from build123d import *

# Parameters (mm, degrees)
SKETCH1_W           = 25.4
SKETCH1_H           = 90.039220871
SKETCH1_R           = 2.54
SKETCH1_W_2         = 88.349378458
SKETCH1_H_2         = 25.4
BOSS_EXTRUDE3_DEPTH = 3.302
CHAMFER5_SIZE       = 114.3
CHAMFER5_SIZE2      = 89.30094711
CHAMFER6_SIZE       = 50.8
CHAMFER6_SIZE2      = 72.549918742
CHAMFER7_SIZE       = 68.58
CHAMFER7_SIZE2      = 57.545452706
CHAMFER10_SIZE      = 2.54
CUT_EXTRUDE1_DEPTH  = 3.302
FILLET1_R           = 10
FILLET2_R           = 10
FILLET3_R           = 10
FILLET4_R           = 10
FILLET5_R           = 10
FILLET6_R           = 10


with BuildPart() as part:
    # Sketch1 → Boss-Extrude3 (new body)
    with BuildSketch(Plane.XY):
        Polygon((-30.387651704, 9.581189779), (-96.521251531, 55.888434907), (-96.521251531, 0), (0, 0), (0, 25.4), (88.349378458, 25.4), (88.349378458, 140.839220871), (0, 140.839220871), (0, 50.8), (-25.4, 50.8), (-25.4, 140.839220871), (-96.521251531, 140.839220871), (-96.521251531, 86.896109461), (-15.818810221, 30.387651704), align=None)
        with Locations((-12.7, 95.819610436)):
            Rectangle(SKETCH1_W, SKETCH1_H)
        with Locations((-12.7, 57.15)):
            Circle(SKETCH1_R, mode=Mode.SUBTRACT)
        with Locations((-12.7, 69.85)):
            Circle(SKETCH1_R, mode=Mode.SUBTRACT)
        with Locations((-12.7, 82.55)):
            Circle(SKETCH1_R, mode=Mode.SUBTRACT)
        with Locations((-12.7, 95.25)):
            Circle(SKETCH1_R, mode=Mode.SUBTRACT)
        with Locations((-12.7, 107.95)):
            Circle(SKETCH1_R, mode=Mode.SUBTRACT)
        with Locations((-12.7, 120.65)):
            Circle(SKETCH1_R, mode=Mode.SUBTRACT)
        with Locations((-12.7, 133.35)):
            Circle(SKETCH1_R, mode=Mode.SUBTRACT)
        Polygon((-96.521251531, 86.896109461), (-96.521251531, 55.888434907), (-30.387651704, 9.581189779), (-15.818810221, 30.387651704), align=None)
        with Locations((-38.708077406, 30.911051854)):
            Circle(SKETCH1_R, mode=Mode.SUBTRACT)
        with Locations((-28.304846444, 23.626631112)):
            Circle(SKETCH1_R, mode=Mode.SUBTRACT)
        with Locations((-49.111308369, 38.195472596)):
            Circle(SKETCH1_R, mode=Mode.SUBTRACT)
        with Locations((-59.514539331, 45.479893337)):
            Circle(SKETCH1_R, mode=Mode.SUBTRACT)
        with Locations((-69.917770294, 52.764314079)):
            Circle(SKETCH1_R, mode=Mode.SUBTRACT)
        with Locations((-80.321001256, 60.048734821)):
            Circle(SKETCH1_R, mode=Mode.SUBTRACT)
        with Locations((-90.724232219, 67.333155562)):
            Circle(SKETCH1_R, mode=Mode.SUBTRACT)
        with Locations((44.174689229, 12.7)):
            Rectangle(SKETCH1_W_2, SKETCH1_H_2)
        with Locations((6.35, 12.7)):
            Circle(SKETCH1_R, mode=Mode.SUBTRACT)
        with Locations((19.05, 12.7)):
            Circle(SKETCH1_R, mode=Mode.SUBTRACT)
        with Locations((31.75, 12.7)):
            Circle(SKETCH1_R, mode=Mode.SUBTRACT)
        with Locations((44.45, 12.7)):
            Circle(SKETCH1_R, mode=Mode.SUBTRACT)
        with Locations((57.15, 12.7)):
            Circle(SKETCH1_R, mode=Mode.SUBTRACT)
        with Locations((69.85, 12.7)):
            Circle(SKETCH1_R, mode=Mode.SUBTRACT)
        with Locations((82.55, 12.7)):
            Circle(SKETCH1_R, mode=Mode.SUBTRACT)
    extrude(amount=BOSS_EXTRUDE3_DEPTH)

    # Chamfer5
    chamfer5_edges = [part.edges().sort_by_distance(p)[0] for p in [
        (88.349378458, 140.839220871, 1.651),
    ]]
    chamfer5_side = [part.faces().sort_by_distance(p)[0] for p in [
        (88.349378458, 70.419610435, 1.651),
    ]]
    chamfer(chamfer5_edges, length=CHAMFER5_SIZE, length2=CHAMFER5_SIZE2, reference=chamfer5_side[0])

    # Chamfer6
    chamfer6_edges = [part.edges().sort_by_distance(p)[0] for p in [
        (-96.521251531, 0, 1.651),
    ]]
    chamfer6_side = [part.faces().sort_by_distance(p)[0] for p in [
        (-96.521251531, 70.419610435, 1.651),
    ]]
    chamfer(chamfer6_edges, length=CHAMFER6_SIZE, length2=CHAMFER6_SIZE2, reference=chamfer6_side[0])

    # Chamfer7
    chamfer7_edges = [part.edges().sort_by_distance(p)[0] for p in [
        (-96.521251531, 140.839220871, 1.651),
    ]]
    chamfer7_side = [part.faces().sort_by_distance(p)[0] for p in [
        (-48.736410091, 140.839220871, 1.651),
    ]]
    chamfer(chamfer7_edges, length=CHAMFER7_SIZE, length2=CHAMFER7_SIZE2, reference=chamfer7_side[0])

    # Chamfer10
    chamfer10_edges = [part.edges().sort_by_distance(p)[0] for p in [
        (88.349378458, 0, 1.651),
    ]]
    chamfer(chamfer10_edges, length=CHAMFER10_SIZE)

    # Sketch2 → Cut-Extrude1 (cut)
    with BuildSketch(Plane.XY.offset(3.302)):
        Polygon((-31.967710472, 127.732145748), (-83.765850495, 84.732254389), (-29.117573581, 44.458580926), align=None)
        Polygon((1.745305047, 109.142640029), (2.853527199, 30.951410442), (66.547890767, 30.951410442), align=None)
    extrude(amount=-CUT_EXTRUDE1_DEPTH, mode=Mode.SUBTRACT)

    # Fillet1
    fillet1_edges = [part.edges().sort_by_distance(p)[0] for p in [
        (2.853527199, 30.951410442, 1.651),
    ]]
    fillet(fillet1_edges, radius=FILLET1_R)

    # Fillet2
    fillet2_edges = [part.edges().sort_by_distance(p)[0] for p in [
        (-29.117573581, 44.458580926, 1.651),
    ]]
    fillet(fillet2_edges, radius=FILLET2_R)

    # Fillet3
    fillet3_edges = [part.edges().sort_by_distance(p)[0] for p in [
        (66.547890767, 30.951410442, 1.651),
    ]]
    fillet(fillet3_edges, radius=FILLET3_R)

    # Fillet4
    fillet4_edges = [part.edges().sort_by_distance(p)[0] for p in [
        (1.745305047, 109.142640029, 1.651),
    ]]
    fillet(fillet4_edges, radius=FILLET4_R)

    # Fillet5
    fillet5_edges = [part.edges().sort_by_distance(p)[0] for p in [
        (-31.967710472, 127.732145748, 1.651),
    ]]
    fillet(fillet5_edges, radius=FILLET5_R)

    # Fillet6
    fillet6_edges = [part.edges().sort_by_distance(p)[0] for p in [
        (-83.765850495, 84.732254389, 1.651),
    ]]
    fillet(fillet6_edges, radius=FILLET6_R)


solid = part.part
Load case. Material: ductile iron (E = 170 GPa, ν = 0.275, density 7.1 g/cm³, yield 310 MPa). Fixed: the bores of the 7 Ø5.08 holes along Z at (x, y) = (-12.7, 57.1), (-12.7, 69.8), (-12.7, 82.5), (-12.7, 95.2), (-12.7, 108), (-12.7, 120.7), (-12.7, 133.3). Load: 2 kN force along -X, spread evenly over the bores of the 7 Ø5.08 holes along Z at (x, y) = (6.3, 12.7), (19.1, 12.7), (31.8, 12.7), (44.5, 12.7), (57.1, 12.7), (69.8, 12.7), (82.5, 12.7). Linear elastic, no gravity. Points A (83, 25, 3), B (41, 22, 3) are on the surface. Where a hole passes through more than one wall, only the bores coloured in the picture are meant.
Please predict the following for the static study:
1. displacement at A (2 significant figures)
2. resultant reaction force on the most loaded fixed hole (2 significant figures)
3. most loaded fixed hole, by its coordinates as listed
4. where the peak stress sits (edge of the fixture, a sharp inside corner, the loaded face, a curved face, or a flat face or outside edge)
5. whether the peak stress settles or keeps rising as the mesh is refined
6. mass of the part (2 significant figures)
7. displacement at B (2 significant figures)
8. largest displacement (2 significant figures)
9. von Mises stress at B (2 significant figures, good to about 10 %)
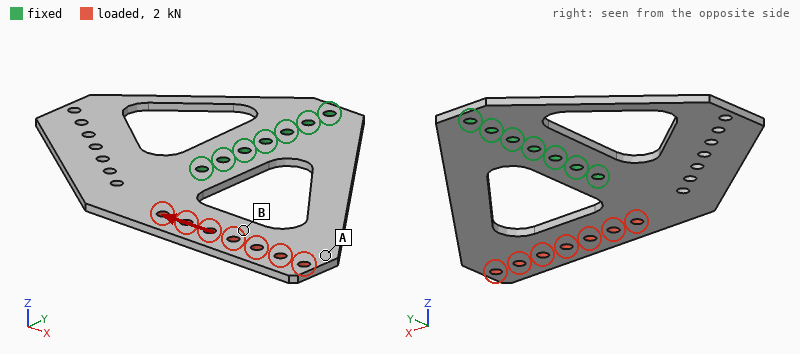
50 µm
3.6 kN
(-12.7, 57.1)
edge of the fixture
keeps rising
290 g
42 µm
55 µm
20 MPa
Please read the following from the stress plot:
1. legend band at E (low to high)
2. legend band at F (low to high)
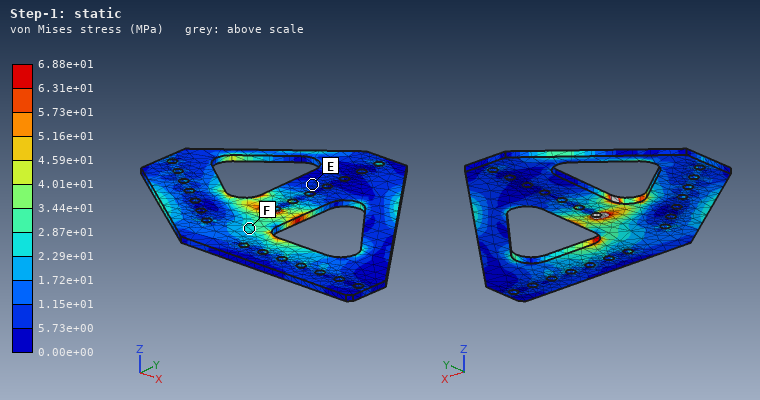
5.73e+00 to 1.15e+01 MPa
2.29e+01 to 2.87e+01 MPa
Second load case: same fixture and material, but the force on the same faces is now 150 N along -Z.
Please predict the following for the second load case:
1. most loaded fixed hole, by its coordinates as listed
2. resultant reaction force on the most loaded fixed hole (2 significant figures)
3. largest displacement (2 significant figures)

(-12.7, 57.1)
290 N
1.6 mm
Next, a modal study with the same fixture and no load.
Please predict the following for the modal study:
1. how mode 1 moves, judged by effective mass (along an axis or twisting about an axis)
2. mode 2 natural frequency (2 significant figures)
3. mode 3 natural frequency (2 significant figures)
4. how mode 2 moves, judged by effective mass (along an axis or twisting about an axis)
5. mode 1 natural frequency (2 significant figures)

along Z
410 Hz
650 Hz
along Z
220 Hz
